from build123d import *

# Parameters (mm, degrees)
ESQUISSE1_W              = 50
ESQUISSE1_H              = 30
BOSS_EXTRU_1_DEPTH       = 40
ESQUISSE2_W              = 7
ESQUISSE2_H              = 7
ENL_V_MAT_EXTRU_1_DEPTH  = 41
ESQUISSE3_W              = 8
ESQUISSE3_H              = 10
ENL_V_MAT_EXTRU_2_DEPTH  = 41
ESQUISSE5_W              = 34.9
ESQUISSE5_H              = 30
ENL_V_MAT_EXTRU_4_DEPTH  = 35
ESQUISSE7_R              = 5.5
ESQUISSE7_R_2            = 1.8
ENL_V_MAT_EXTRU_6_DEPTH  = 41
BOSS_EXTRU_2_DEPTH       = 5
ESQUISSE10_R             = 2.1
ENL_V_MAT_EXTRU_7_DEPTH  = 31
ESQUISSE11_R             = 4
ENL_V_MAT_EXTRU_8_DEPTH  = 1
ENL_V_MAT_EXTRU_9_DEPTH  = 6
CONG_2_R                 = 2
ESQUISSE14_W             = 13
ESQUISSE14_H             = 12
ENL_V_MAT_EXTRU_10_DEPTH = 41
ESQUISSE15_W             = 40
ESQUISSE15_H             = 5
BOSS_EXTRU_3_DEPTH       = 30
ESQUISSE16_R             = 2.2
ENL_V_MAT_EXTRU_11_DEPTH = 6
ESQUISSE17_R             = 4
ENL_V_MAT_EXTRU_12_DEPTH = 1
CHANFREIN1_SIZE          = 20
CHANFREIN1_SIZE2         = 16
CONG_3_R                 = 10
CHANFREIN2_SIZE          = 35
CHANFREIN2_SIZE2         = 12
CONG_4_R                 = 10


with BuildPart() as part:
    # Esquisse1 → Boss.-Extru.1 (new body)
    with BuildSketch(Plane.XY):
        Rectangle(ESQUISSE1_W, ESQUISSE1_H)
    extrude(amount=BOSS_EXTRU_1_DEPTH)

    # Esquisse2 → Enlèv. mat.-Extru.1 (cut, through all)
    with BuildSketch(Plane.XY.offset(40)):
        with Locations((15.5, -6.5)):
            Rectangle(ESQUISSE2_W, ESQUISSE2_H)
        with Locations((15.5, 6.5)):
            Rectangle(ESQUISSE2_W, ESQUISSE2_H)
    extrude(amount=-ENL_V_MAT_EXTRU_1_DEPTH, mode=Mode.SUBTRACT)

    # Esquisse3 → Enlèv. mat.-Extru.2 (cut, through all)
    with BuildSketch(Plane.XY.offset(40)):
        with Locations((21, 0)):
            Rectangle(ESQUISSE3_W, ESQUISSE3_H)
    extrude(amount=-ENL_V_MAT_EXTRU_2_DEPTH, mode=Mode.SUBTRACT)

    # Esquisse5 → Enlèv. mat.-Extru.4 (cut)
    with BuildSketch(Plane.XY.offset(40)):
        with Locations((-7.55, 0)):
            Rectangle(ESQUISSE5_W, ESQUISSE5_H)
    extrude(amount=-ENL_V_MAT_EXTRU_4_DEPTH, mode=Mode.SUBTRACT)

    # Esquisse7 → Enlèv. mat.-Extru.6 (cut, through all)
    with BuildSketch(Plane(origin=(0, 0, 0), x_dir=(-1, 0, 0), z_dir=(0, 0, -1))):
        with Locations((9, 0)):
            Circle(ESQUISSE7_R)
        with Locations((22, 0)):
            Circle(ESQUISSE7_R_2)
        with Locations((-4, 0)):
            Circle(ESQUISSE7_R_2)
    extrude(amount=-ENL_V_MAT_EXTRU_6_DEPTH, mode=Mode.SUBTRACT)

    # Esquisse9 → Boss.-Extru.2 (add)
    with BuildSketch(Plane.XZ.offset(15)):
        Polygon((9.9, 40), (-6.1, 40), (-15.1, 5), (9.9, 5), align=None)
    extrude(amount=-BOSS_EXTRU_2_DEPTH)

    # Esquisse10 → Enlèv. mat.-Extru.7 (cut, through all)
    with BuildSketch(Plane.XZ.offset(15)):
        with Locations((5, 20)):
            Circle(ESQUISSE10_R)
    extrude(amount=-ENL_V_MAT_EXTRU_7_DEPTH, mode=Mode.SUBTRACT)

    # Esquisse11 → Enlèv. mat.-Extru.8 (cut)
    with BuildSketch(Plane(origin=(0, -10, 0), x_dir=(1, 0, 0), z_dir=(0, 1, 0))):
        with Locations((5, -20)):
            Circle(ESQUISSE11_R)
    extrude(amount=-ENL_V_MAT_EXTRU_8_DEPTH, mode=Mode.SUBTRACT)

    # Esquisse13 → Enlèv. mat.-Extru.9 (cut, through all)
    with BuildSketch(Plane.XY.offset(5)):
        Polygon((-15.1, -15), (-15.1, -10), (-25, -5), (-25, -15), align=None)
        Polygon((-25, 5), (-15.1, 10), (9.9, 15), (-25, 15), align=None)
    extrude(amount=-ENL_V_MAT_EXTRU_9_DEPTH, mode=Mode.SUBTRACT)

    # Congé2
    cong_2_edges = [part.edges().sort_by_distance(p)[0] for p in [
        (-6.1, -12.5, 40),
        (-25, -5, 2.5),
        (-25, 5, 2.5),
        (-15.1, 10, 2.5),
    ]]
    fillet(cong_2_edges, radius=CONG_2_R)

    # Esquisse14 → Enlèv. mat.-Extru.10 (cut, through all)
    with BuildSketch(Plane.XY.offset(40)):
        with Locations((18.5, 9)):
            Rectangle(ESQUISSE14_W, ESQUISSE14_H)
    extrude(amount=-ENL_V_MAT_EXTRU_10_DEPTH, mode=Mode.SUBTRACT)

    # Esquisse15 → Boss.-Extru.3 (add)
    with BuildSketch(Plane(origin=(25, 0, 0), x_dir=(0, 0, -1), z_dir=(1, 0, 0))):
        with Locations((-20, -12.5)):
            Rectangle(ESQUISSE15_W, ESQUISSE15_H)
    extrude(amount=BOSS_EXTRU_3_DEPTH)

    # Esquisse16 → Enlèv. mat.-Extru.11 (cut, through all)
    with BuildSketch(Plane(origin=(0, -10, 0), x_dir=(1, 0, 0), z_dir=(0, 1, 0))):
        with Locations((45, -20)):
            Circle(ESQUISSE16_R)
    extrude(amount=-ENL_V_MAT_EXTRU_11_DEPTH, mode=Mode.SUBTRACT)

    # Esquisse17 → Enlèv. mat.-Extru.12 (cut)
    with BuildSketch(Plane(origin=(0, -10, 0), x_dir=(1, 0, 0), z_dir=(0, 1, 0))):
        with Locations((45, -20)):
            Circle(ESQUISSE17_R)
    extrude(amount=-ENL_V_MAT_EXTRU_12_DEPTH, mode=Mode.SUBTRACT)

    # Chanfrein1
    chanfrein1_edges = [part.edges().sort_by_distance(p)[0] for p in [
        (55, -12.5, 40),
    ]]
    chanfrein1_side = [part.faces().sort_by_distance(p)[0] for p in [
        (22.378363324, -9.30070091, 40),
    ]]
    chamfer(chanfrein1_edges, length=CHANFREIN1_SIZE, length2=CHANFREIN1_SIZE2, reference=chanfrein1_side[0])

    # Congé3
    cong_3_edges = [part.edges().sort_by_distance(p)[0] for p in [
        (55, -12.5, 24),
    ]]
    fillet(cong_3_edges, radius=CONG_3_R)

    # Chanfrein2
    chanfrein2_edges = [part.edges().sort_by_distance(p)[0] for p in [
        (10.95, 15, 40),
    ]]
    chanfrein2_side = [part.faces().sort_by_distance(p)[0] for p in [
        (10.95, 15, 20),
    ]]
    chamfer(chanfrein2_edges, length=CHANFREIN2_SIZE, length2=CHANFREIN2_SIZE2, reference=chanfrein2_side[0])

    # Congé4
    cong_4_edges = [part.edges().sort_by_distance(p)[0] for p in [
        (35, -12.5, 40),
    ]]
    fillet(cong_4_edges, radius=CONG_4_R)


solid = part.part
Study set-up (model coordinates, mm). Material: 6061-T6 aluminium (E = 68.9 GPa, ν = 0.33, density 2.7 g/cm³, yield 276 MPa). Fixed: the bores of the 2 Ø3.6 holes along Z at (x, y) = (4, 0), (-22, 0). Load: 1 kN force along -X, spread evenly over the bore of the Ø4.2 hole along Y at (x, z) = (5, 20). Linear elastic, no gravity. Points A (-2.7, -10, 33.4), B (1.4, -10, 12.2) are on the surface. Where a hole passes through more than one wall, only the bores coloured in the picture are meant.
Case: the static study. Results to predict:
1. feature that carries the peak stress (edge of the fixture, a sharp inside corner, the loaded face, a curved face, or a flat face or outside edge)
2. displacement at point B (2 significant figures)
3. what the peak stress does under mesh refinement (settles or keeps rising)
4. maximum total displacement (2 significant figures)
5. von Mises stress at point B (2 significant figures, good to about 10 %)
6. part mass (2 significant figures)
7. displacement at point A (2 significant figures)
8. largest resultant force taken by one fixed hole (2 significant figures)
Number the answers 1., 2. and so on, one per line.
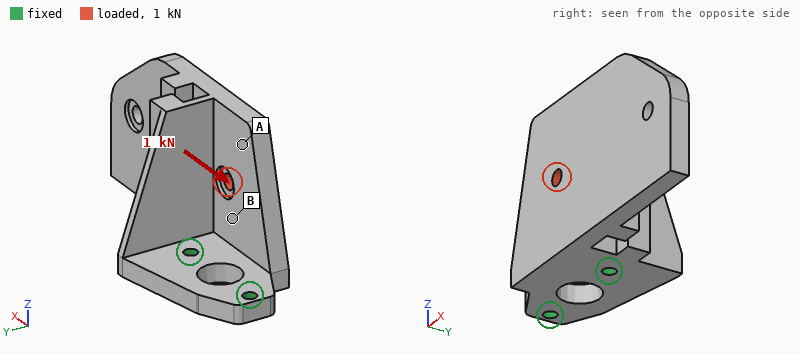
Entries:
1. edge of the fixture
2. 0.033 mm
3. keeps rising
4. 0.17 mm
5. 22 MPa
6. 52 g
7. 0.097 mm
8. 920 N
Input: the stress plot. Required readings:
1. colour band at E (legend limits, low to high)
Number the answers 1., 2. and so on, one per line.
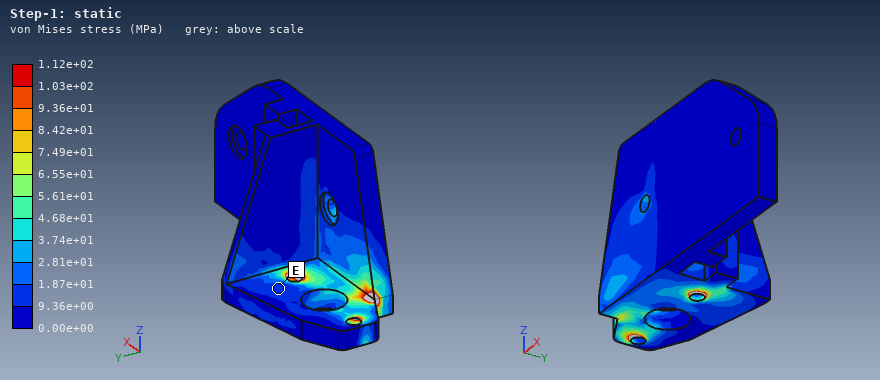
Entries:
1. 9.36e+00 to 1.87e+01 MPa
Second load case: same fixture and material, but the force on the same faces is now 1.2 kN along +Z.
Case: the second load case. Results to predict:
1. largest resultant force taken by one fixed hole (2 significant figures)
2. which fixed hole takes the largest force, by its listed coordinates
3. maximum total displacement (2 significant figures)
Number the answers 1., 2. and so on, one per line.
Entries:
1. 1.1 kN
2. (4, 0)
3. 0.17 mm
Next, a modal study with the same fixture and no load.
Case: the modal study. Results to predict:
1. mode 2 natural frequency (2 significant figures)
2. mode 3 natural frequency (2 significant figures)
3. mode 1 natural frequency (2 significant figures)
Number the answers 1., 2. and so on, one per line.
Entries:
1. 2000 Hz
2. 2900 Hz
3. 1400 Hz
